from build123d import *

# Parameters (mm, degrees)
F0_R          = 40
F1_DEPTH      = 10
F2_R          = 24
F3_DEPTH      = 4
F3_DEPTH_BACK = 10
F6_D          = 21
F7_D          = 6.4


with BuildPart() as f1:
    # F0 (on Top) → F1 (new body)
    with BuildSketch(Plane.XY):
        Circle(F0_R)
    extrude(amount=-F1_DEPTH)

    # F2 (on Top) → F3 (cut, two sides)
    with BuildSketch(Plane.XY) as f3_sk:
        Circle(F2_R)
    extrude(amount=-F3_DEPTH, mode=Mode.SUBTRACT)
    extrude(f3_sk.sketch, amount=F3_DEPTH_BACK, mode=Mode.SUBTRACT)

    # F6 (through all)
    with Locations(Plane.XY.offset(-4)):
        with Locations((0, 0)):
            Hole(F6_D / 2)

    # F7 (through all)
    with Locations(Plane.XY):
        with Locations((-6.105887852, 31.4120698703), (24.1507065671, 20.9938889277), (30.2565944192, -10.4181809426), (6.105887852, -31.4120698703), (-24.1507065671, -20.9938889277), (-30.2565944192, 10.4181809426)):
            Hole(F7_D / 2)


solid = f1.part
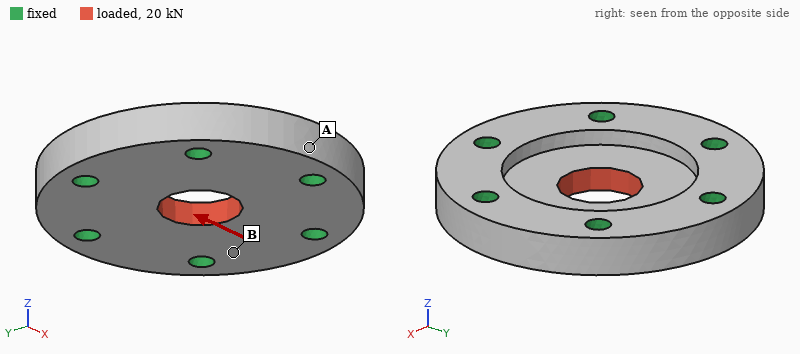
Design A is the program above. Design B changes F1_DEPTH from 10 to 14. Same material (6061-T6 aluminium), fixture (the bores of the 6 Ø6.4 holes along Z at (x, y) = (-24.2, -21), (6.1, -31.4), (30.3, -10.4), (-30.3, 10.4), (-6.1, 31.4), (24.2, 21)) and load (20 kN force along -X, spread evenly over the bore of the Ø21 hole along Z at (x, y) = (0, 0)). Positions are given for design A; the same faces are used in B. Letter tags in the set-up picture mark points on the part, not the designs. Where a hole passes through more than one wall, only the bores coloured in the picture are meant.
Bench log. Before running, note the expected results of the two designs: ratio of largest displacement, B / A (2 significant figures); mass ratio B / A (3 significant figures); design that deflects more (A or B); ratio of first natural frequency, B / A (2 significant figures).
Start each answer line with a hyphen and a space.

- 0.61
- 1.46
- A
- 1.2
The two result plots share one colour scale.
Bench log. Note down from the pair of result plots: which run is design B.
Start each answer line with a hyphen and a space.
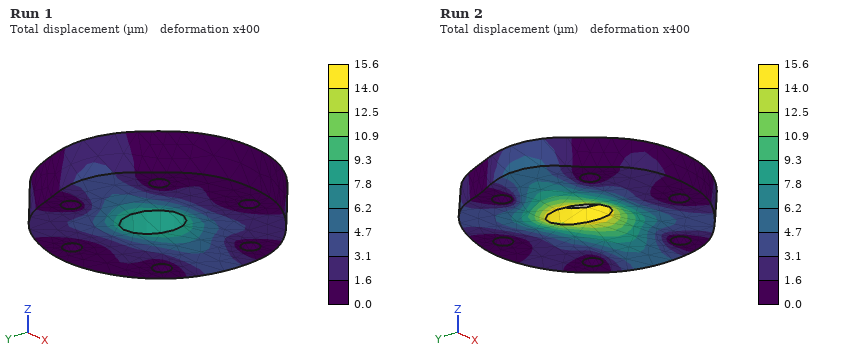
- Run 1
